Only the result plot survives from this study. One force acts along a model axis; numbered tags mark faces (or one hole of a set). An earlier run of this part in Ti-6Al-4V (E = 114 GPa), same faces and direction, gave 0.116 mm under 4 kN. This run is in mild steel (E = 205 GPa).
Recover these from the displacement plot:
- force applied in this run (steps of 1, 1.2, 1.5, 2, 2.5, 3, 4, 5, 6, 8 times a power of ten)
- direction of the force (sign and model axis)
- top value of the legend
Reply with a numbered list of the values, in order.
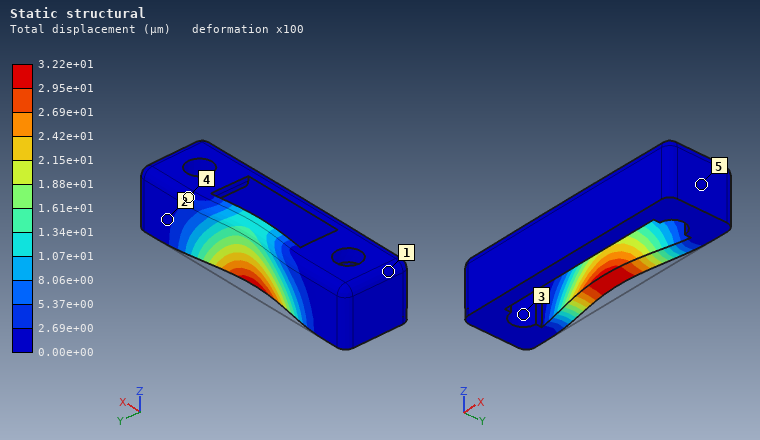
1. 2 kN
2. -Y
3. 3.22e+01 µm
